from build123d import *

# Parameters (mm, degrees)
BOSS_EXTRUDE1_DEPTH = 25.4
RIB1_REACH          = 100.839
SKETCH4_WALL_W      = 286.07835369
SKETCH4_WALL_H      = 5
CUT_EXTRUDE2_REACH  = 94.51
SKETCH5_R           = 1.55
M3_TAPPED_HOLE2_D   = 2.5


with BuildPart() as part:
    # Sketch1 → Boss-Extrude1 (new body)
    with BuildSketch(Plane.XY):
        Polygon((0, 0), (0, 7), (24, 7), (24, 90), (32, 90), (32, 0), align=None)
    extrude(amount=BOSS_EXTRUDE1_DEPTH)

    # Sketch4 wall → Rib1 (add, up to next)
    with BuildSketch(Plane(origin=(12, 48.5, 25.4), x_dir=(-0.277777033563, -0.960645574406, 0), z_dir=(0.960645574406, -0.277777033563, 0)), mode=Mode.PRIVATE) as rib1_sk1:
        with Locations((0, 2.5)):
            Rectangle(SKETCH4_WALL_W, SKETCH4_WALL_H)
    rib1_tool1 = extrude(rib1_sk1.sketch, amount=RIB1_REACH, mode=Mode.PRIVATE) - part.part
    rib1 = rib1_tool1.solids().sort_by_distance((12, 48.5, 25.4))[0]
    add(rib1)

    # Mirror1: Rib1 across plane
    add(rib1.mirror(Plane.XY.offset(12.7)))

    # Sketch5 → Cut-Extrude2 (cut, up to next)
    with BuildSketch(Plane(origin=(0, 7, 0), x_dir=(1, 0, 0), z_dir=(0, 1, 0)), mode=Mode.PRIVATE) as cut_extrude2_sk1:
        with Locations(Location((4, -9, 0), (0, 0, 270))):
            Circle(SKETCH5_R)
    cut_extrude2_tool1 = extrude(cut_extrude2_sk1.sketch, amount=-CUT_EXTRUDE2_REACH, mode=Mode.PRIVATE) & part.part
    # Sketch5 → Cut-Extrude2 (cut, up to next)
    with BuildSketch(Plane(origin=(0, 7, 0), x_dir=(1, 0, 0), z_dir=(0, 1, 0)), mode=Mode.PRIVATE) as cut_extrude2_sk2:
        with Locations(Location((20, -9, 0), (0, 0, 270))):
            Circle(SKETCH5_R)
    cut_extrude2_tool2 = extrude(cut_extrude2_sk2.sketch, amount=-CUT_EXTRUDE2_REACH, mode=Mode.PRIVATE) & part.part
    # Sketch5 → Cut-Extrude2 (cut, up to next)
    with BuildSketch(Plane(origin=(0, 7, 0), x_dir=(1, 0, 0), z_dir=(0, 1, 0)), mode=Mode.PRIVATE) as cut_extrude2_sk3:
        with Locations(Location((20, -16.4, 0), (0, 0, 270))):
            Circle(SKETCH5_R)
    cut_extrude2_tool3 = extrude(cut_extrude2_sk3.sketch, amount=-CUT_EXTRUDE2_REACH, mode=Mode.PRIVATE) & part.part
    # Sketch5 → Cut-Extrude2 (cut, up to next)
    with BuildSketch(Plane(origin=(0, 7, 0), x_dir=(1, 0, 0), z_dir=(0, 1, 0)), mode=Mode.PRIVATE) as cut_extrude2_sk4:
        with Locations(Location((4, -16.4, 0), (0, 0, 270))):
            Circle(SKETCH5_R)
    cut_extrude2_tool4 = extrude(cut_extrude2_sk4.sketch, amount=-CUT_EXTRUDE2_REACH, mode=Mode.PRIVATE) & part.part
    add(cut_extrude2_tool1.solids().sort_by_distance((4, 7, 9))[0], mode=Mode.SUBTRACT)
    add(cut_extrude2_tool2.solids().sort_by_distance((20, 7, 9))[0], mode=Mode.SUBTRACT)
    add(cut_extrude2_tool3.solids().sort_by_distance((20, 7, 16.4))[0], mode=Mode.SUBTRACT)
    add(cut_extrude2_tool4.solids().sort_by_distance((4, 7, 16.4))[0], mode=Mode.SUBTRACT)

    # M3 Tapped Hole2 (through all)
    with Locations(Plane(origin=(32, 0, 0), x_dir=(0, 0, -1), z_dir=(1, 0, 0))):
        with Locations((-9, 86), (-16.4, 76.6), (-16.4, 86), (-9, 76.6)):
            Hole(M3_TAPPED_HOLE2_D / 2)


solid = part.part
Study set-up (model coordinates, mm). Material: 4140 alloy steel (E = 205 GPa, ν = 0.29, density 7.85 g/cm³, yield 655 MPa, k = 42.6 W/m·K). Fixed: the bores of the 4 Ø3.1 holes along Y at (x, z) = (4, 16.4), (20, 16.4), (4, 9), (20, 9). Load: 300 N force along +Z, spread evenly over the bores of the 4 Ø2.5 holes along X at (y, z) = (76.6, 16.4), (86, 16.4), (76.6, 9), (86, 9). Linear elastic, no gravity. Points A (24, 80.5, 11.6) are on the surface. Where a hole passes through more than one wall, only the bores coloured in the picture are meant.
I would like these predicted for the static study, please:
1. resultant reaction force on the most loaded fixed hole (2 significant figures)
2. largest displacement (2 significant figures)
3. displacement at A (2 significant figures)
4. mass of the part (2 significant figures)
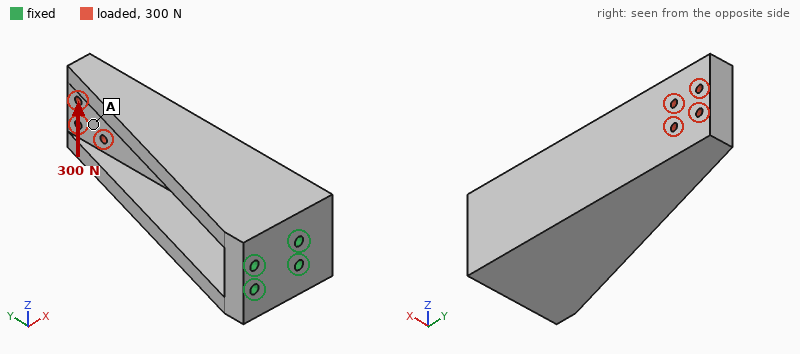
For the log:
1.1 kN
32 µm
28 µm
250 g
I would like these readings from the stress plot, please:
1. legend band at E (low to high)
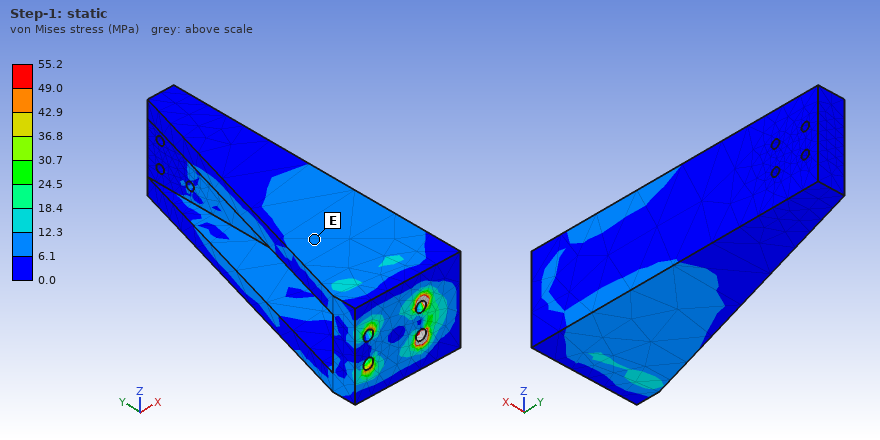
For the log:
6.1 to 12.3 MPa
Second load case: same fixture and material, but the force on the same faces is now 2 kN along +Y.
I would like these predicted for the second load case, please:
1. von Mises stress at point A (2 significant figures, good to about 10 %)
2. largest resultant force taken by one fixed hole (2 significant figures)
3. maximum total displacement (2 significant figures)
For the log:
7.5 MPa
1.2 kN
22 µm
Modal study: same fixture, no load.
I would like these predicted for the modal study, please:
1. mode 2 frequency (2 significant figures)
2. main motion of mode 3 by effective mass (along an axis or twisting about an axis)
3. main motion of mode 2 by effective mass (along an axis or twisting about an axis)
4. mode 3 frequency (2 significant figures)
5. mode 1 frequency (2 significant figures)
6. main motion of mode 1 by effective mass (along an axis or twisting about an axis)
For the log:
2500 Hz
twisting about Y
along X
6400 Hz
1900 Hz
along Z
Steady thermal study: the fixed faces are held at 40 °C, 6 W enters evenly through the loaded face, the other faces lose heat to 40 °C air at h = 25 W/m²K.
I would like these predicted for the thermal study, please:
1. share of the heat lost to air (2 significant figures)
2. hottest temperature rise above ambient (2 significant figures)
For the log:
45 %
27 K
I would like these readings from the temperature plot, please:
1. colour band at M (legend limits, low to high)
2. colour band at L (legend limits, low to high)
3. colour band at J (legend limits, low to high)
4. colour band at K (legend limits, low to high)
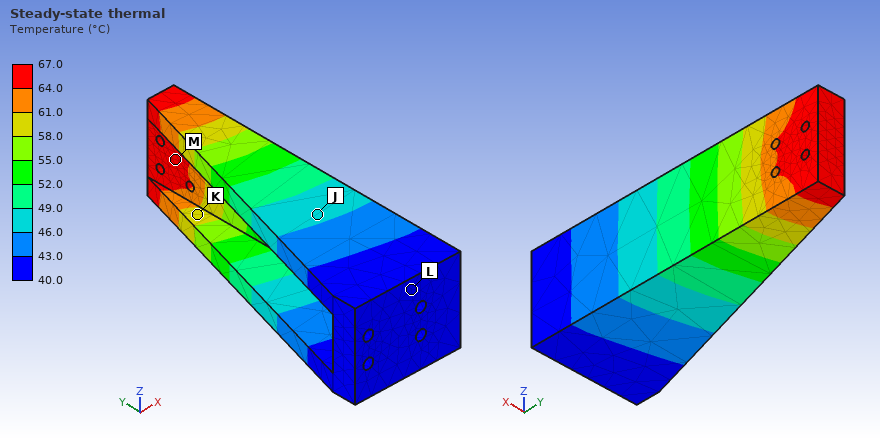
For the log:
64.0 to 67.0 °C
40.0 to 43.0 °C
46.0 to 49.0 °C
58.0 to 61.0 °C
